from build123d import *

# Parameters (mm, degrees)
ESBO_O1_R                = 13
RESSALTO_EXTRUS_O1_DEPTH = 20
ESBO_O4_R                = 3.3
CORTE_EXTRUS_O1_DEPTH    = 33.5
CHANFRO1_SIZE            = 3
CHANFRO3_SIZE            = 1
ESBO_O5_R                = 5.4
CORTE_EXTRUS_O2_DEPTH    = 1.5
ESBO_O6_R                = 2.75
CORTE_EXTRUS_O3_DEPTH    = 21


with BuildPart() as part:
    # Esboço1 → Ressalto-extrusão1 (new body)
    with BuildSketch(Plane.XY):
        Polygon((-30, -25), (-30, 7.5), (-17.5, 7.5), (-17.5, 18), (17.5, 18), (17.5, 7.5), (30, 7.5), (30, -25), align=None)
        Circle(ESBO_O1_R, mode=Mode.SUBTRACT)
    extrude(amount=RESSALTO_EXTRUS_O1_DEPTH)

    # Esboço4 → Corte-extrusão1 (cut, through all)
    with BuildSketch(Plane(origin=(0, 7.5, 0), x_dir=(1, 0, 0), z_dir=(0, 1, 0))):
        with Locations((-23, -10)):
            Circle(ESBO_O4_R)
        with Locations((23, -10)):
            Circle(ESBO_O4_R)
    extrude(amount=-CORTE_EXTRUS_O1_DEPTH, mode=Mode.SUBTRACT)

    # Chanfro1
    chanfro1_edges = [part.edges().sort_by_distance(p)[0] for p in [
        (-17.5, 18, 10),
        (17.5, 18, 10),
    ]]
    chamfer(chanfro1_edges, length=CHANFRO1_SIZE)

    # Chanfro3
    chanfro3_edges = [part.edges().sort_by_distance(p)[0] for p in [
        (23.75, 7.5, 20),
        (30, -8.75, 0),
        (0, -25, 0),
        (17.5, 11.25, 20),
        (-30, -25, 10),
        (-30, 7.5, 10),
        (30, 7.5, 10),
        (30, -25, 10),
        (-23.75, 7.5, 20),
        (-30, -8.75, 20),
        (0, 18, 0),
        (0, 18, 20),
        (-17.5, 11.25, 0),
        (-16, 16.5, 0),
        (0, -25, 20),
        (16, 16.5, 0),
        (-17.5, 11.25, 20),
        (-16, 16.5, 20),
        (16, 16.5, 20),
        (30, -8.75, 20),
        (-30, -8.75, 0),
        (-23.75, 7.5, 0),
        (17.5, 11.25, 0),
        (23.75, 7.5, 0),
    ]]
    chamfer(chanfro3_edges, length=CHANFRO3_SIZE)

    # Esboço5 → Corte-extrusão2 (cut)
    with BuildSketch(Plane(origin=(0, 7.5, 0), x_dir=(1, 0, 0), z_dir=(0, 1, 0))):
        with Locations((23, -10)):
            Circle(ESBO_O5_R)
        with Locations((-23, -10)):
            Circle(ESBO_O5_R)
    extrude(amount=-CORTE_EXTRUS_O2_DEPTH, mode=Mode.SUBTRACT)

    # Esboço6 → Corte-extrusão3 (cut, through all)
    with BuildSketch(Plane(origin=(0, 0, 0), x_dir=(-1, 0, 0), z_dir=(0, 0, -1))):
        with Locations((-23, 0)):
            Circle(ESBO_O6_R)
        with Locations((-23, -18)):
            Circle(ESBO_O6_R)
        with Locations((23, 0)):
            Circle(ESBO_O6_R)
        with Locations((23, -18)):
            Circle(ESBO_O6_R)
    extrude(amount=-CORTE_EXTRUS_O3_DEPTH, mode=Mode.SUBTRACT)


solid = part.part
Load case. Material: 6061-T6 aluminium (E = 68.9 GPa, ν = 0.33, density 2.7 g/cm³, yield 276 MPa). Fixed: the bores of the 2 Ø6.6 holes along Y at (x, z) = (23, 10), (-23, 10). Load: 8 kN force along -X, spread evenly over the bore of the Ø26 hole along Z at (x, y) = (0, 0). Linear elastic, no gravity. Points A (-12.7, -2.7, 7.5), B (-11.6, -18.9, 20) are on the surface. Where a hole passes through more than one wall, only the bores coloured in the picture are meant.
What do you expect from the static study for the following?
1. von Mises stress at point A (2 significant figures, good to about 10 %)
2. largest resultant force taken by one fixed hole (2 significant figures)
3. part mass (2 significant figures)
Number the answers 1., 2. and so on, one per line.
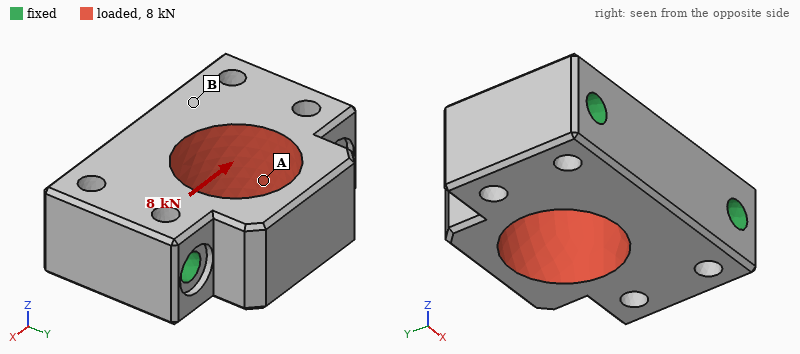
1. 13 MPa
2. 4.0 kN
3. 85 g
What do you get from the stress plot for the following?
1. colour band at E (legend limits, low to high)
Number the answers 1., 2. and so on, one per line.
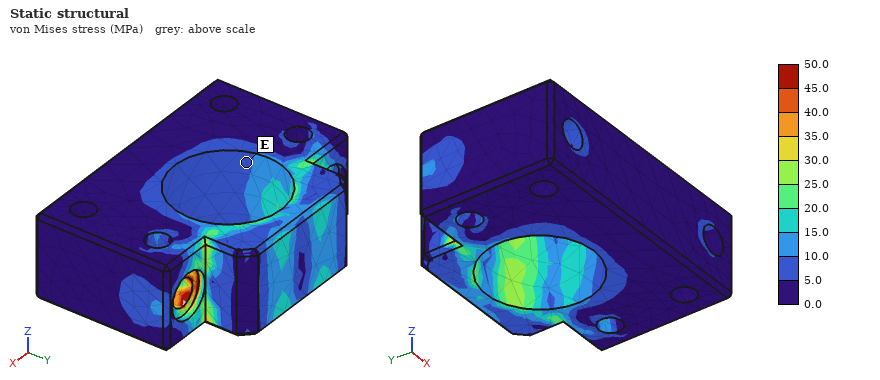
1. 5.0 to 10.0 MPa
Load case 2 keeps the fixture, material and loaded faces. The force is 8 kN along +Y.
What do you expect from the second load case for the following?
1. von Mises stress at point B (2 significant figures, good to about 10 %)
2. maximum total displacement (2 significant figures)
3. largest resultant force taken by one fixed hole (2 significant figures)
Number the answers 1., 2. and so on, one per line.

1. 6.9 MPa
2. 9.9 µm
3. 4.1 kN
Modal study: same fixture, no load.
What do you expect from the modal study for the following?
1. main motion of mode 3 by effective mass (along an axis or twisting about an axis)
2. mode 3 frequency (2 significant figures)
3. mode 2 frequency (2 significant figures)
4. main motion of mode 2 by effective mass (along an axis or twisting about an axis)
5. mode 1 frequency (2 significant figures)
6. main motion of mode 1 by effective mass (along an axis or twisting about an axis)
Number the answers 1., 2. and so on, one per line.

1. along Z
2. 26 kHz
3. 23 kHz
4. along X
5. 16 kHz
6. along Z
